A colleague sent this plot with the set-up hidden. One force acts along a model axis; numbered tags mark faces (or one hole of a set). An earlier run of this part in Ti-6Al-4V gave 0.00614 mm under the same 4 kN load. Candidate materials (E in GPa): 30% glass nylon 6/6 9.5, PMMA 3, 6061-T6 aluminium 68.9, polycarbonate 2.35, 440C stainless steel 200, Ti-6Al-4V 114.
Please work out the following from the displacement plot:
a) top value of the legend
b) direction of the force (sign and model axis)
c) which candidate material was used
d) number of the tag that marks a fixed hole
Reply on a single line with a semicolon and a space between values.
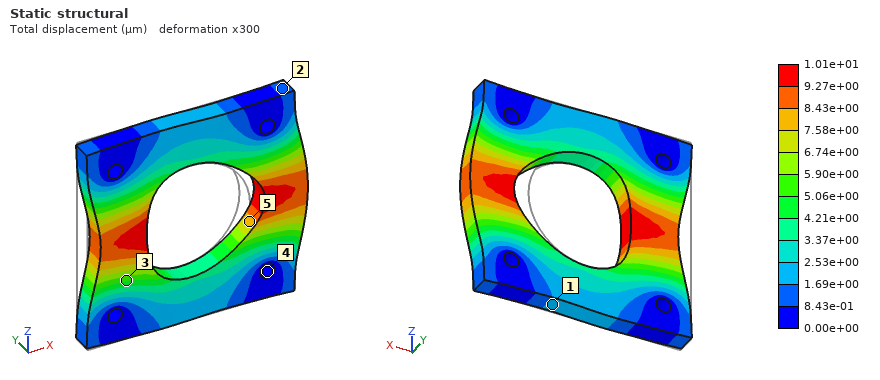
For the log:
1.01e+01 µm; +X; 6061-T6 aluminium; 4
